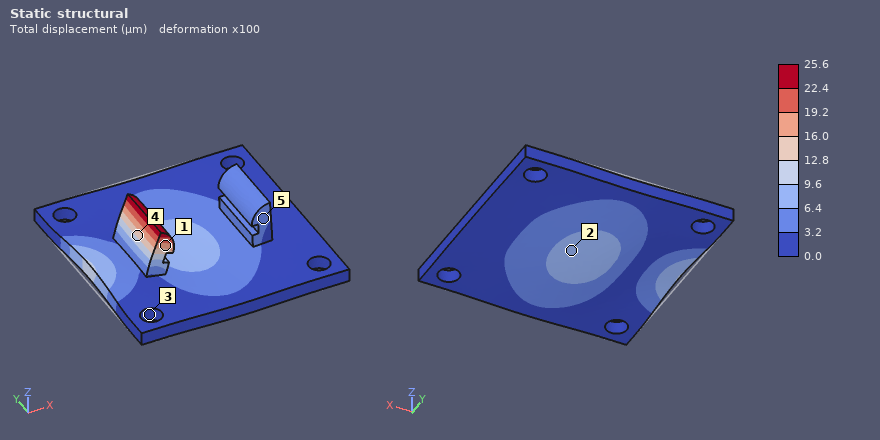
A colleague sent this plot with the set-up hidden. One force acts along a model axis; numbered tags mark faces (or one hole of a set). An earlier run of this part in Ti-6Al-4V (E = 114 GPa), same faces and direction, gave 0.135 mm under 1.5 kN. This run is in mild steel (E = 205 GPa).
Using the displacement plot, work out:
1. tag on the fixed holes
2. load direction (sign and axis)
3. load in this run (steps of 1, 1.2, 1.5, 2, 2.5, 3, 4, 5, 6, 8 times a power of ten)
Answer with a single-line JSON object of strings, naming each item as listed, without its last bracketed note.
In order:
{"tag on the fixed holes": "3", "load direction": "+X", "load in this run": "500 N"}
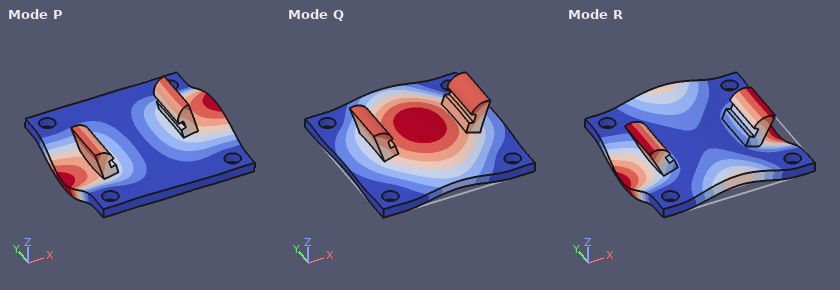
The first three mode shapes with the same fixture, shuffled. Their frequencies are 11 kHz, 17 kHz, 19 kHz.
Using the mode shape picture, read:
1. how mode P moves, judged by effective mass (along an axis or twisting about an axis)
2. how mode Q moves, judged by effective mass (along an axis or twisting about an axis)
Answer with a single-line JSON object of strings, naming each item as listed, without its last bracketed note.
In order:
{"how mode P moves, judged by effective mass": "twisting about Y", "how mode Q moves, judged by effective mass": "along Z"}
